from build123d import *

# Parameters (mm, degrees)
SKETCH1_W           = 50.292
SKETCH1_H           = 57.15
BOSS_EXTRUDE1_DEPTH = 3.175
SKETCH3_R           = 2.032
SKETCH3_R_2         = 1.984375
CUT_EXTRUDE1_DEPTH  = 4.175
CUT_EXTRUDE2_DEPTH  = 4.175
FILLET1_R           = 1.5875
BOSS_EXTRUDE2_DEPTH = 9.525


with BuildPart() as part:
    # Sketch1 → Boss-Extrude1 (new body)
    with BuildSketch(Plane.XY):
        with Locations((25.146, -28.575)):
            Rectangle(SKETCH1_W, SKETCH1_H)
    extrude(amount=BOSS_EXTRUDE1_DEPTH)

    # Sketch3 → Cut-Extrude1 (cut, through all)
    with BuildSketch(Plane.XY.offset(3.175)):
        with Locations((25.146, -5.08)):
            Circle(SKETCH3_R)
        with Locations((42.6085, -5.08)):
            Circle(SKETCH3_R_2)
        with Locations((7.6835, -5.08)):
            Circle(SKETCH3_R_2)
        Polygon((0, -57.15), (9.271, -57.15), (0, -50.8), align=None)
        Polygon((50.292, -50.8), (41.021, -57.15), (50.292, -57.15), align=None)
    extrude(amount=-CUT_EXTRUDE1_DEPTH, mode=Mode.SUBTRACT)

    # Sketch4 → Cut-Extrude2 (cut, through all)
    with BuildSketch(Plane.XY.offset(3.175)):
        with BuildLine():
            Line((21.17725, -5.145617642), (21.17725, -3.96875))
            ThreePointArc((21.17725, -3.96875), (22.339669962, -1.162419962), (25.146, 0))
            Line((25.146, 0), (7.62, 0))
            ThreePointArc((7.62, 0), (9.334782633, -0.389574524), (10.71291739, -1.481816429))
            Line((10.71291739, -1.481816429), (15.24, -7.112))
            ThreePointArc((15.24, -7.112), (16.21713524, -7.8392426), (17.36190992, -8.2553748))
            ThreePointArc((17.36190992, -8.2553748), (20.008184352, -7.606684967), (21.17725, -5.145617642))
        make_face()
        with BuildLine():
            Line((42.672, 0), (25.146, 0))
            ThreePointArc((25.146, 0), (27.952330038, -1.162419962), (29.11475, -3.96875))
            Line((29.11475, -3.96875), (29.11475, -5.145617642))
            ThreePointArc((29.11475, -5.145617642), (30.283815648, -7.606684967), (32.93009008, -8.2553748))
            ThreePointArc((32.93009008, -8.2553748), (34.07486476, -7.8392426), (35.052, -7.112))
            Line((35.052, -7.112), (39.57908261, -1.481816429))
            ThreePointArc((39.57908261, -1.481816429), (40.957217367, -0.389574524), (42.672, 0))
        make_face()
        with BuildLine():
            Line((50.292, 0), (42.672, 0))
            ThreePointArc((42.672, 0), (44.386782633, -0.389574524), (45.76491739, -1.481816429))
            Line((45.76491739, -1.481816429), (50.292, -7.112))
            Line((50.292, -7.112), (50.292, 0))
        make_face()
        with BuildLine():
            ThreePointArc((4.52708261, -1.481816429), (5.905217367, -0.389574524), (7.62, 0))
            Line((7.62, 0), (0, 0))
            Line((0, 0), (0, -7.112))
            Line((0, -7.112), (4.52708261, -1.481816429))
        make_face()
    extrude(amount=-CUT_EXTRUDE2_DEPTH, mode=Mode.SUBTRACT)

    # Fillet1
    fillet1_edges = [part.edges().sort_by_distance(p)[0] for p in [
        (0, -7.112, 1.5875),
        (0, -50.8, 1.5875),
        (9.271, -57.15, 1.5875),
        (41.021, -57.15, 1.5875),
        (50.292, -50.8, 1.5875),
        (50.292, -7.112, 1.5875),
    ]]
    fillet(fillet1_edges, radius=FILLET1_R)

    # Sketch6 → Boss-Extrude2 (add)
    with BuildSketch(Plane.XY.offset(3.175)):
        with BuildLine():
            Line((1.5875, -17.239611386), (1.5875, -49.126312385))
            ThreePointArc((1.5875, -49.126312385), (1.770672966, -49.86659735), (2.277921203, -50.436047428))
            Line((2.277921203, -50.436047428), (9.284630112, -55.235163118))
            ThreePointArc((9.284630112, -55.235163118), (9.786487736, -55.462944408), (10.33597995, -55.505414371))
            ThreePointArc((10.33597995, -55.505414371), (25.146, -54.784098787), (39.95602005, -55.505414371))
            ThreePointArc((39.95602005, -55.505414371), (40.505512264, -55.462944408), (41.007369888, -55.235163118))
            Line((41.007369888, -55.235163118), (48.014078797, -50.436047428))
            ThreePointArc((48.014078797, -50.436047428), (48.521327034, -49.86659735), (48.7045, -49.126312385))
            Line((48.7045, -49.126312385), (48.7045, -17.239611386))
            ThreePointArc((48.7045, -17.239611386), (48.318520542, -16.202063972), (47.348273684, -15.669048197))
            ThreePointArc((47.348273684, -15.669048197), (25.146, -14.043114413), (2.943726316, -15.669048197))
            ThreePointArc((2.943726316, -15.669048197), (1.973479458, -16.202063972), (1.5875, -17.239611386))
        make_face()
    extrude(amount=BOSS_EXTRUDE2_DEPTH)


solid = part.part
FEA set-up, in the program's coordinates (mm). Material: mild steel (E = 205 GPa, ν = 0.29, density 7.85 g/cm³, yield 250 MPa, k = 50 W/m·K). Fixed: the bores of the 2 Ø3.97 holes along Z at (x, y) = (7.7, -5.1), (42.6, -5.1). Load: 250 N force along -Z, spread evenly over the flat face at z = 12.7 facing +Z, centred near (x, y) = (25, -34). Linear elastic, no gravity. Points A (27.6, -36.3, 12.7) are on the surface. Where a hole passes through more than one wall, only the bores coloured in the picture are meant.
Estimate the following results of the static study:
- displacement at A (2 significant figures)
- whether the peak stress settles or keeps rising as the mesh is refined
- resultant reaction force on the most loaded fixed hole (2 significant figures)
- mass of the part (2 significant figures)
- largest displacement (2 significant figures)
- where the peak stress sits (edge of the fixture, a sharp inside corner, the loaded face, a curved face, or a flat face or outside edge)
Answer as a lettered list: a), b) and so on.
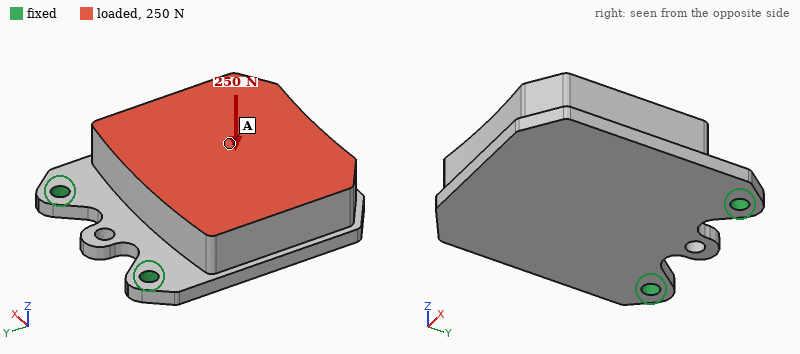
a) 0.097 mm
b) keeps rising
c) 130 N
d) 200 g
e) 0.16 mm
f) edge of the fixture
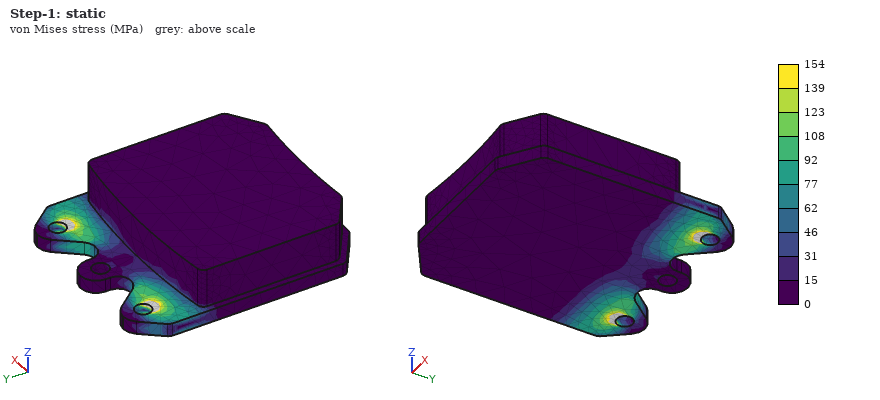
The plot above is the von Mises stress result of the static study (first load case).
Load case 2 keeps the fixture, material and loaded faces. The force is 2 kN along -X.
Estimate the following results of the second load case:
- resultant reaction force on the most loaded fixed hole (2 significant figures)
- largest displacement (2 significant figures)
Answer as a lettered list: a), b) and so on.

a) 1.9 kN
b) 22 µm
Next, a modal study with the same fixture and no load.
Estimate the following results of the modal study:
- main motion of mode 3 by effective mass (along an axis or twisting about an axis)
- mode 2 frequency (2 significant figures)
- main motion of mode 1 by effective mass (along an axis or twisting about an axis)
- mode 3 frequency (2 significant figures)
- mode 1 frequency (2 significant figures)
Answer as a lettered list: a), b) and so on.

a) along X
b) 4200 Hz
c) along Z
d) 5500 Hz
e) 550 Hz
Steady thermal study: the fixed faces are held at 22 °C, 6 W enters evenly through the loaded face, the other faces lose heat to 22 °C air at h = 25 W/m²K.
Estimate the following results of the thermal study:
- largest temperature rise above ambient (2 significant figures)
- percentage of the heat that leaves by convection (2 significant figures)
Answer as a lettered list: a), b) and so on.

a) 14 K
b) 25 %
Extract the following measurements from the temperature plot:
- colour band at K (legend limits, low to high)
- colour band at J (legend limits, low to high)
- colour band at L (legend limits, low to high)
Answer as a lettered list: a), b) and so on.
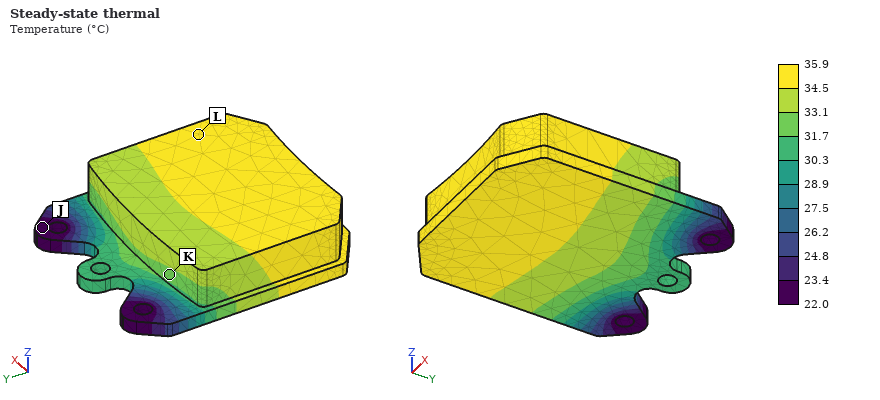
a) 31.7 to 33.1 °C
b) 22.0 to 23.4 °C
c) 34.5 to 35.9 °C
